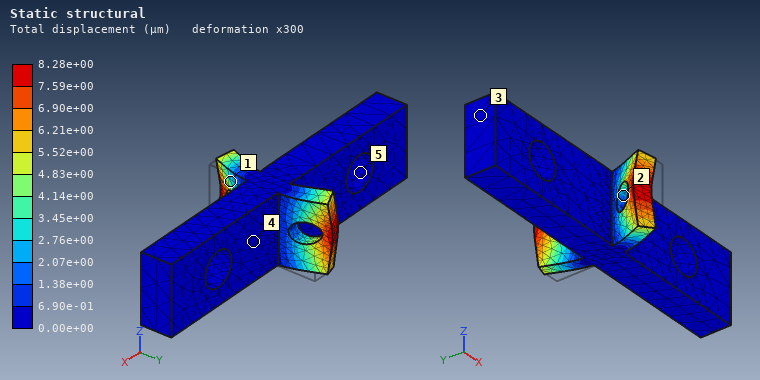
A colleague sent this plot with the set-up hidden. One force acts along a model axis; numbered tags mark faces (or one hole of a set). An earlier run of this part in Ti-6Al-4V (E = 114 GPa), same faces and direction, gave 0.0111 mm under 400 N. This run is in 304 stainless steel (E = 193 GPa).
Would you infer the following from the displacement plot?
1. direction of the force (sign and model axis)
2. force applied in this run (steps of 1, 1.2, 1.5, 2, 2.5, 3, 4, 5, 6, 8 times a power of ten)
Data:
-X
500 N
